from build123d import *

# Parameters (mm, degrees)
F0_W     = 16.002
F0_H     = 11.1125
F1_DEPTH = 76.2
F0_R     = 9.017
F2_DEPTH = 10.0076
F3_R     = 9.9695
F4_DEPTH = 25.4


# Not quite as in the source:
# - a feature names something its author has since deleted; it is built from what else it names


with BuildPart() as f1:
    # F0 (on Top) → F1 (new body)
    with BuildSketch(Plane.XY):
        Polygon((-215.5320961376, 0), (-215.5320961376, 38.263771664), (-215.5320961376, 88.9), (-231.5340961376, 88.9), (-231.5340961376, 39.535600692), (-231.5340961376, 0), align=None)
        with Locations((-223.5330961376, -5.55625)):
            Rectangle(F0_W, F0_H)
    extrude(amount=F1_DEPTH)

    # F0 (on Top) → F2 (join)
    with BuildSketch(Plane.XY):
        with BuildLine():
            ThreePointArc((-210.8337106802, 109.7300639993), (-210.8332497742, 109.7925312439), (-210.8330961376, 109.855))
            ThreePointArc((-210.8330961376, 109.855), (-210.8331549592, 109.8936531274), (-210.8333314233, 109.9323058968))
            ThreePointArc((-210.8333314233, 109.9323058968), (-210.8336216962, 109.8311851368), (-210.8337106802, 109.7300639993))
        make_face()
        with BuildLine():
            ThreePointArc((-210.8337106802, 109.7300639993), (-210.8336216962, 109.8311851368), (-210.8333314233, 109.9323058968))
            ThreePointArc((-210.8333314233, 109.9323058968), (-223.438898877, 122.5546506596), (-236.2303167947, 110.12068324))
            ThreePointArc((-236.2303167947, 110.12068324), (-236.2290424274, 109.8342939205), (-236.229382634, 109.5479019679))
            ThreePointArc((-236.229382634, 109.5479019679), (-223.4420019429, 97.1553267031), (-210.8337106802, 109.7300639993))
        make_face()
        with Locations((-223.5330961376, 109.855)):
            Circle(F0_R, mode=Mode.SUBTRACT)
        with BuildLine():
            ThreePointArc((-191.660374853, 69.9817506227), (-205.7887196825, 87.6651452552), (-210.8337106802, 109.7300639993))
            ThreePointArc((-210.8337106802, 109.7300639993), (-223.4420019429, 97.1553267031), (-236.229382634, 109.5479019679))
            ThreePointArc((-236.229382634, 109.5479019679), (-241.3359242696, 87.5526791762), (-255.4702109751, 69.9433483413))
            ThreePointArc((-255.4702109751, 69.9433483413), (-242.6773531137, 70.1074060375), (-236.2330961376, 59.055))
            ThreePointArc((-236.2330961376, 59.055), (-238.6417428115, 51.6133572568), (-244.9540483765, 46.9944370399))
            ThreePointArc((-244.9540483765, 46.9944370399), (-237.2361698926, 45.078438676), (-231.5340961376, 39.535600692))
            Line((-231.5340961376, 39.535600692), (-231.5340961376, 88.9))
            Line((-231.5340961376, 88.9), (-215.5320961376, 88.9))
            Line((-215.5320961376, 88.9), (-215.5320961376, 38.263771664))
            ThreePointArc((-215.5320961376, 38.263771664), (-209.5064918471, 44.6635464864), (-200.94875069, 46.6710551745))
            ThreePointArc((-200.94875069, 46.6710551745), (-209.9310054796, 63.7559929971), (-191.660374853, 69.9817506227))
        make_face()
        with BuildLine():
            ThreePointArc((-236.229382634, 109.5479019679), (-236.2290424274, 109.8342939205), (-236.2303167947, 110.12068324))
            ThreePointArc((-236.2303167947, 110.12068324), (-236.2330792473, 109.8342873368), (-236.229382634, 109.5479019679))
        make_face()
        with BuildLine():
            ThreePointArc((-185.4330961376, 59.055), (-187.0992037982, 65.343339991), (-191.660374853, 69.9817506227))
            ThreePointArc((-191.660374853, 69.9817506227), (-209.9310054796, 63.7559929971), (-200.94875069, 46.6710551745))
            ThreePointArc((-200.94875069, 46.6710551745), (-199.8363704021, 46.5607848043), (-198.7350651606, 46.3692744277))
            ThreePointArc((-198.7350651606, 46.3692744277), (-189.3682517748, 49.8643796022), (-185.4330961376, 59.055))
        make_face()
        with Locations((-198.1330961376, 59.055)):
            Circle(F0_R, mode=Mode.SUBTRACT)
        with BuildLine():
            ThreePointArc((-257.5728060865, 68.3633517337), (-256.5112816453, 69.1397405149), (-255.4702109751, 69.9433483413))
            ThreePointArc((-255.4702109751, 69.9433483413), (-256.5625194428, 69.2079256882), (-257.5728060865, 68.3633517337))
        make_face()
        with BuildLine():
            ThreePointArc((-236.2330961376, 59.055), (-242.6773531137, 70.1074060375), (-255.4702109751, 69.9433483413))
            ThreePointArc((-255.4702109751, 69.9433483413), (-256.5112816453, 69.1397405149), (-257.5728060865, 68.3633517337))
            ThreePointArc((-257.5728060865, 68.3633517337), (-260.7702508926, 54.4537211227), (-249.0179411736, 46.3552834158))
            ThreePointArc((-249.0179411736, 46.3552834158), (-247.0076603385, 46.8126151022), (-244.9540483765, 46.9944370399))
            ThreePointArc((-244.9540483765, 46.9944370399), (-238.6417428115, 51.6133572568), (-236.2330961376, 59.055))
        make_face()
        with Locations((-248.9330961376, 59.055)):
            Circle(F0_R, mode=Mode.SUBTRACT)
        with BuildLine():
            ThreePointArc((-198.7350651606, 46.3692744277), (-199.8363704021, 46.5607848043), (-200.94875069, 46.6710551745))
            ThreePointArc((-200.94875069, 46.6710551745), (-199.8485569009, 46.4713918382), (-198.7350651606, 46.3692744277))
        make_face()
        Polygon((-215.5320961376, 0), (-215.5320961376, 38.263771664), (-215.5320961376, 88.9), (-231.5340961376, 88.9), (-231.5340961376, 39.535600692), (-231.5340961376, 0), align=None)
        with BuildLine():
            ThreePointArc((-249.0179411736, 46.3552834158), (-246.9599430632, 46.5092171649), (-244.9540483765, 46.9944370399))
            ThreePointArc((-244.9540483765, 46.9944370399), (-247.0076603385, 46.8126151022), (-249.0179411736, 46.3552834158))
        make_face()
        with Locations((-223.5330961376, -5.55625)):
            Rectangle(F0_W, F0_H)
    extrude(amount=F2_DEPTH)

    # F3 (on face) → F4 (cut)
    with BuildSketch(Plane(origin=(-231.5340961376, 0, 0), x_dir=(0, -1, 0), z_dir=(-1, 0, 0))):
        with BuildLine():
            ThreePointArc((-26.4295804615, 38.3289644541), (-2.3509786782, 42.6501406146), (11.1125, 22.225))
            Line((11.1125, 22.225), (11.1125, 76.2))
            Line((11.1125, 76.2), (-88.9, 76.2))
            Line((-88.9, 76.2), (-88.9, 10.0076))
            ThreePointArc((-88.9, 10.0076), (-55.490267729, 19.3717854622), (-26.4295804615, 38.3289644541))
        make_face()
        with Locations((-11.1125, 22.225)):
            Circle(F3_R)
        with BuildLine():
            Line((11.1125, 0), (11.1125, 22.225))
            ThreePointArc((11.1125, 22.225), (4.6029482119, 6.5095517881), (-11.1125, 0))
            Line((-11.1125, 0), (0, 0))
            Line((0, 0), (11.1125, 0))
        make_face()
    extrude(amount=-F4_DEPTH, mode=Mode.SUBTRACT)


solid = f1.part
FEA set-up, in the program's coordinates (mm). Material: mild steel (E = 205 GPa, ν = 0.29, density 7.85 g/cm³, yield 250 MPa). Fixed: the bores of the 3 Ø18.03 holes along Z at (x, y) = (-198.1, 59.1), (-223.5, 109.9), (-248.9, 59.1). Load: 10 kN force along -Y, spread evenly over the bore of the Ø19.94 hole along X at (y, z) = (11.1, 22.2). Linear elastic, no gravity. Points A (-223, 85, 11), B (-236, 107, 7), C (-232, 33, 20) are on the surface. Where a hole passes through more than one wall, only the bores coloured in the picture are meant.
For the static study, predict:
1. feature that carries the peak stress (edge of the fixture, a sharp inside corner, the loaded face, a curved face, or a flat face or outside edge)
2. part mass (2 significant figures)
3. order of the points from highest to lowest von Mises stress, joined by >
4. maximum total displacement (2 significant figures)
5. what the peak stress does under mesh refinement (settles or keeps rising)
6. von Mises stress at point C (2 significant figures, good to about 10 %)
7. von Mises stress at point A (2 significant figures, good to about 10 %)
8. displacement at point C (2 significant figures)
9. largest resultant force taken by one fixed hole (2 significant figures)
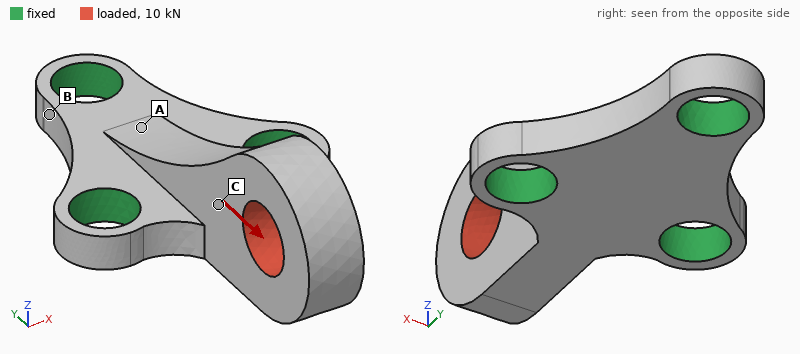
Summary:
edge of the fixture
460 g
A > C > B
0.12 mm
keeps rising
29 MPa
42 MPa
0.042 mm
3.7 kN
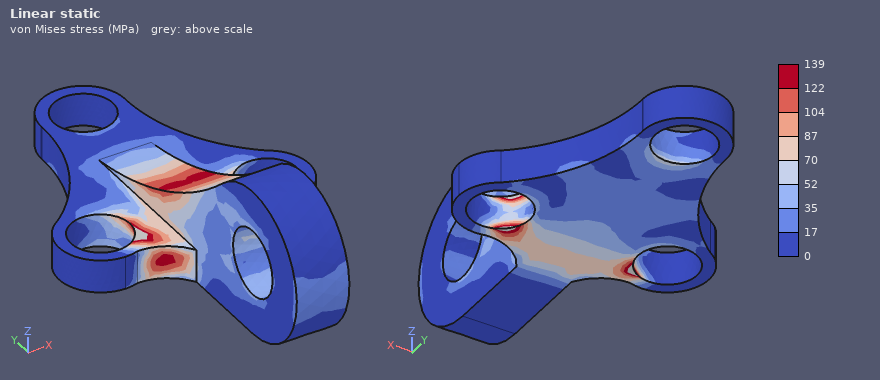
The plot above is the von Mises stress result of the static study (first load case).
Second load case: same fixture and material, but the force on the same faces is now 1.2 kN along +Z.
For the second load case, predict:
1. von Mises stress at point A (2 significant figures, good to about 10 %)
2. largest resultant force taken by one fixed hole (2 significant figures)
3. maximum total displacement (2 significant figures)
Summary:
9.9 MPa
1.1 kN
42 µm
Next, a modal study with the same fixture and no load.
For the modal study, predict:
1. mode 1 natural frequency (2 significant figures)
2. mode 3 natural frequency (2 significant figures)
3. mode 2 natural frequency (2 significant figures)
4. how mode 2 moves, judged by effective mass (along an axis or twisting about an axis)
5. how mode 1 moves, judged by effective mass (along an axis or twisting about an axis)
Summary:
2300 Hz
6600 Hz
2800 Hz
along X
along Z
